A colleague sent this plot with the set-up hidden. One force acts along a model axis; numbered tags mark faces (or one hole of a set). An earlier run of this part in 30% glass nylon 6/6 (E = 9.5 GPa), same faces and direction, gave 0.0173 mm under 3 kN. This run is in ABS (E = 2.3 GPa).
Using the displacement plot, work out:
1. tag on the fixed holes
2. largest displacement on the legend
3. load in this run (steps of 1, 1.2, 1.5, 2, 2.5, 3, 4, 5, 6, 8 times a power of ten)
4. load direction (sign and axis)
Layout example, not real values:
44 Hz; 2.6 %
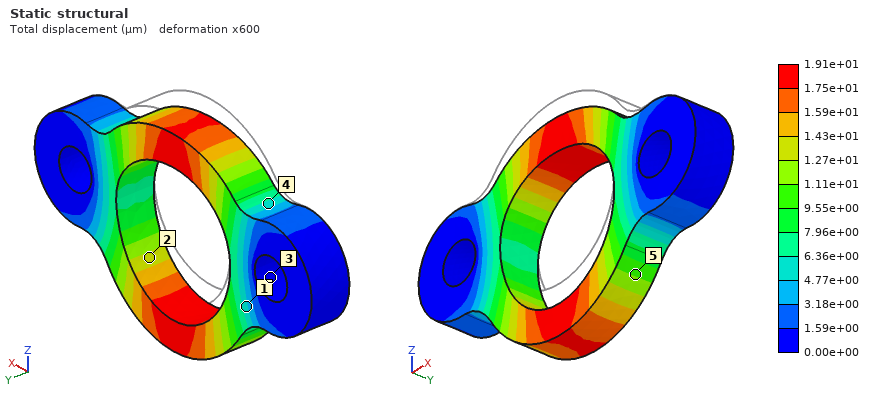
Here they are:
3; 1.91e+01 µm; 800 N; -Z
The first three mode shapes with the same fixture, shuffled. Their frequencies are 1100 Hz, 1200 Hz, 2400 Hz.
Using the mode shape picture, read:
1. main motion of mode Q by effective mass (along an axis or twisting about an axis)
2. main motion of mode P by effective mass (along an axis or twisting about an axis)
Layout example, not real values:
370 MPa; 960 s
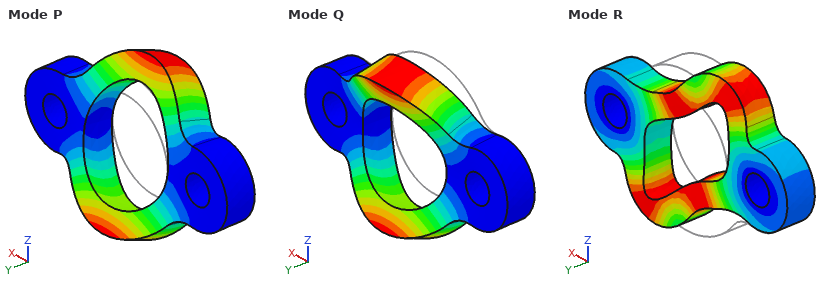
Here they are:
along Y; twisting about X
